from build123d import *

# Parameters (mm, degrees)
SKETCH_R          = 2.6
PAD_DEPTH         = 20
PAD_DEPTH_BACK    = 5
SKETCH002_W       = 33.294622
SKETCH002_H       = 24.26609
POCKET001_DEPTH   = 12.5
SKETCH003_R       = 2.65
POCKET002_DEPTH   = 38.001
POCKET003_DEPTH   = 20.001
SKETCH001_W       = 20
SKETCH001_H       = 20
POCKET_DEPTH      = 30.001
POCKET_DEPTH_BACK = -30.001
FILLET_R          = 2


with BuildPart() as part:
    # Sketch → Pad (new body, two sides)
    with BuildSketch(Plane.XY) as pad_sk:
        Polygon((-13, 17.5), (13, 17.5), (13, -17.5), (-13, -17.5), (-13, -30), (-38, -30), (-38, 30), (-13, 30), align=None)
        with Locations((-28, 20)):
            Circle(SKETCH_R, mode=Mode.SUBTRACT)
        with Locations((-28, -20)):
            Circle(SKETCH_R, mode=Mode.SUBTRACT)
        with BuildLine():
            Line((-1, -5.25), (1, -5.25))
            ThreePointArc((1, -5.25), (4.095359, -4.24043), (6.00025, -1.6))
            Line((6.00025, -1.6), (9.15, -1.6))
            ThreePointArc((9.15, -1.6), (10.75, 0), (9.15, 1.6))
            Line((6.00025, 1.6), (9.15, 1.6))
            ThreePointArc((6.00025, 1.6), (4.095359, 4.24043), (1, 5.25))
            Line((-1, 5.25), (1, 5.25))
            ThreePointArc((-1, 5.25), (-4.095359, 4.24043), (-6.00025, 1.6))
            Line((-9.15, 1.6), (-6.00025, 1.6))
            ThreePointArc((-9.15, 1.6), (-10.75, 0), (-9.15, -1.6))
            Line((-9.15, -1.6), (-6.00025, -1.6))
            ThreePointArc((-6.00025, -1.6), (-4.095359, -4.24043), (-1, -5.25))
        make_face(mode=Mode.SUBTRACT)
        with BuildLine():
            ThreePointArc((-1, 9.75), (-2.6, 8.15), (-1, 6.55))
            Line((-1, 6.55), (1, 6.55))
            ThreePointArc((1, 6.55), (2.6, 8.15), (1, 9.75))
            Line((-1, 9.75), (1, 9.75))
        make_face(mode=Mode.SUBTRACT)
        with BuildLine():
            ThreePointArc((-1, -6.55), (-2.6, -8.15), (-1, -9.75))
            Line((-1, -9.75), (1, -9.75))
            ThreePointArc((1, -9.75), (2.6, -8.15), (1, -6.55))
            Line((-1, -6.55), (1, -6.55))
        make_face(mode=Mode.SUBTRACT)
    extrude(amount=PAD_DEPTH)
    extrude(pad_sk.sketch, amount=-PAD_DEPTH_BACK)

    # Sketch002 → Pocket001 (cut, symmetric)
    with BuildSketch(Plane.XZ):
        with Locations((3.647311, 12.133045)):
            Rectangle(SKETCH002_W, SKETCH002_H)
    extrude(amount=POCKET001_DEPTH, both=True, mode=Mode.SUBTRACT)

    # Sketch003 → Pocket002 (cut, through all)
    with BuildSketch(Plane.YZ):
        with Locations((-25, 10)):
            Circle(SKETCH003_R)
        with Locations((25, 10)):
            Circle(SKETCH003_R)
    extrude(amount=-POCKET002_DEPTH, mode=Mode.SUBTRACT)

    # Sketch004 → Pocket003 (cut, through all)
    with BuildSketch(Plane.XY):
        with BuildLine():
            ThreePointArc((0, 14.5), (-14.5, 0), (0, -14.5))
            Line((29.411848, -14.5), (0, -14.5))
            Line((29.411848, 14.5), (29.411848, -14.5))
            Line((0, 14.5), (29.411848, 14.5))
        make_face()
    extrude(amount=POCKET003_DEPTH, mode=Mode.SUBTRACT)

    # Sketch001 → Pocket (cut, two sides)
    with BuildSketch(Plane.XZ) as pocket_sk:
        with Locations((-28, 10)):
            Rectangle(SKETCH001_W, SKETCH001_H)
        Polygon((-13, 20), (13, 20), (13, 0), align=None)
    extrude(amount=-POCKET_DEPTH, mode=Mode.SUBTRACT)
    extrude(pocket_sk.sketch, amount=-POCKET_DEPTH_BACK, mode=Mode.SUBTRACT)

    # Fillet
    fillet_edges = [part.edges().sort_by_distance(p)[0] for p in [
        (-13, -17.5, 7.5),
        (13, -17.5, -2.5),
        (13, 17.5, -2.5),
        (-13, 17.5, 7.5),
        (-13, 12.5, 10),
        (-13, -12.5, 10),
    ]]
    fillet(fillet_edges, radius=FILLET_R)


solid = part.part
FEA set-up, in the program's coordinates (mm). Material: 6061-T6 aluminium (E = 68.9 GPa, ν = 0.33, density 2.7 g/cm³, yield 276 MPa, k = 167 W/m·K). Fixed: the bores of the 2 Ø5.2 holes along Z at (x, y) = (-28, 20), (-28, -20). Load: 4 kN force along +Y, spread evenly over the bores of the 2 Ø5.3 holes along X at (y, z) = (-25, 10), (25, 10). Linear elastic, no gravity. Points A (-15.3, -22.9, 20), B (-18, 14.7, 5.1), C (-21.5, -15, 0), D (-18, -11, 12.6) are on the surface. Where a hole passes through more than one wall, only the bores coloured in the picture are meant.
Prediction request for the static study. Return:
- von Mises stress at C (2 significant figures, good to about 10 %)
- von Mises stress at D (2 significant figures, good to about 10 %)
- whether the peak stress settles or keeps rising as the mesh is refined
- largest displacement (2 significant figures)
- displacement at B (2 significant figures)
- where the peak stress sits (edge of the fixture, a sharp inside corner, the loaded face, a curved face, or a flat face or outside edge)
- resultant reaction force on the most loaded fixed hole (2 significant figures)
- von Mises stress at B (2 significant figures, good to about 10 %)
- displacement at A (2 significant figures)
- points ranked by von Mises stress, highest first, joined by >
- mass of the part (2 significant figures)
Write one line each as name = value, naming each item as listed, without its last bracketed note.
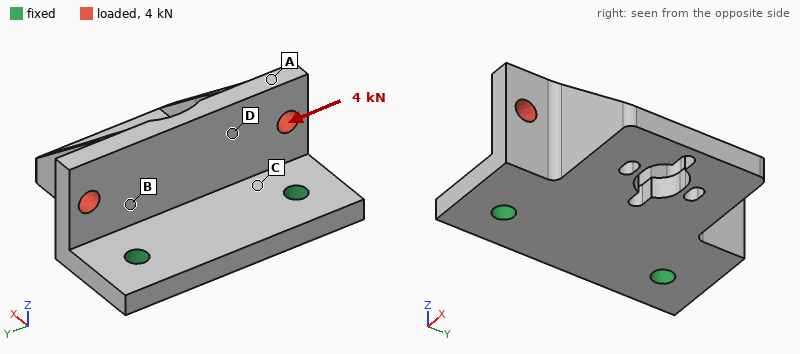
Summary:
von Mises stress at C = 62 MPa
von Mises stress at D = 23 MPa
whether the peak stress settles or keeps rising as the mesh is refined = keeps rising
largest displacement = 71 µm
displacement at B = 29 µm
where the peak stress sits = edge of the fixture
resultant reaction force on the most loaded fixed hole = 2.5 kN
von Mises stress at B = 44 MPa
displacement at A = 63 µm
points ranked by von Mises stress, highest first, joined by > = C > B > D > A
mass of the part = 51 g
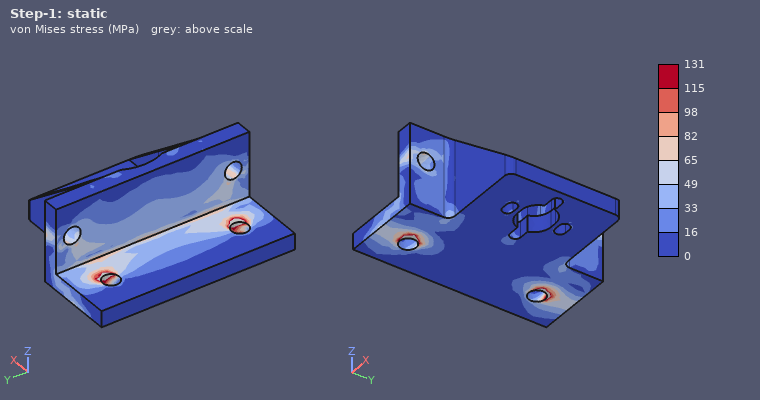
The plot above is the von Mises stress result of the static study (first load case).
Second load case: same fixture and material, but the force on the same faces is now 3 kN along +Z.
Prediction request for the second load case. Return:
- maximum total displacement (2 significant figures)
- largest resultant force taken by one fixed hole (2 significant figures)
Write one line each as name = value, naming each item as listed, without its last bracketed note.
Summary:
maximum total displacement = 0.22 mm
largest resultant force taken by one fixed hole = 1.5 kN
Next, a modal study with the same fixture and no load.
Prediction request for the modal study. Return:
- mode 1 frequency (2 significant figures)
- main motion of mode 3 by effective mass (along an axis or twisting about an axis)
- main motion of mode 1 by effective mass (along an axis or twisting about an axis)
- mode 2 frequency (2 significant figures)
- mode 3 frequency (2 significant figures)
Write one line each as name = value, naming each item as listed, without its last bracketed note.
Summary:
mode 1 frequency = 2500 Hz
main motion of mode 3 by effective mass = along Y
main motion of mode 1 by effective mass = along Z
mode 2 frequency = 6000 Hz
mode 3 frequency = 11 kHz
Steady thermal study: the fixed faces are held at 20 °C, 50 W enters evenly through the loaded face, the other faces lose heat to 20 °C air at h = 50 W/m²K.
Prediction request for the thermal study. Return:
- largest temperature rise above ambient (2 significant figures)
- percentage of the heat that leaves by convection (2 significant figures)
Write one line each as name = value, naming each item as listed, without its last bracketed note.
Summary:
largest temperature rise above ambient = 34 K
percentage of the heat that leaves by convection = 12 %
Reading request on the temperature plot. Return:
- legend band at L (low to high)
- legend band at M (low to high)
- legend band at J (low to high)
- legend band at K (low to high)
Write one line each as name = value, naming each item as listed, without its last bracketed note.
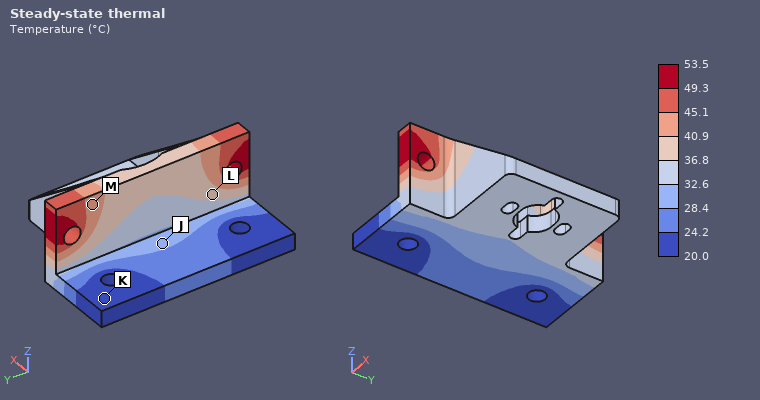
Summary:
legend band at L = 36.8 to 40.9 °C
legend band at M = 40.9 to 45.1 °C
legend band at J = 28.4 to 32.6 °C
legend band at K = 20.0 to 24.2 °C
